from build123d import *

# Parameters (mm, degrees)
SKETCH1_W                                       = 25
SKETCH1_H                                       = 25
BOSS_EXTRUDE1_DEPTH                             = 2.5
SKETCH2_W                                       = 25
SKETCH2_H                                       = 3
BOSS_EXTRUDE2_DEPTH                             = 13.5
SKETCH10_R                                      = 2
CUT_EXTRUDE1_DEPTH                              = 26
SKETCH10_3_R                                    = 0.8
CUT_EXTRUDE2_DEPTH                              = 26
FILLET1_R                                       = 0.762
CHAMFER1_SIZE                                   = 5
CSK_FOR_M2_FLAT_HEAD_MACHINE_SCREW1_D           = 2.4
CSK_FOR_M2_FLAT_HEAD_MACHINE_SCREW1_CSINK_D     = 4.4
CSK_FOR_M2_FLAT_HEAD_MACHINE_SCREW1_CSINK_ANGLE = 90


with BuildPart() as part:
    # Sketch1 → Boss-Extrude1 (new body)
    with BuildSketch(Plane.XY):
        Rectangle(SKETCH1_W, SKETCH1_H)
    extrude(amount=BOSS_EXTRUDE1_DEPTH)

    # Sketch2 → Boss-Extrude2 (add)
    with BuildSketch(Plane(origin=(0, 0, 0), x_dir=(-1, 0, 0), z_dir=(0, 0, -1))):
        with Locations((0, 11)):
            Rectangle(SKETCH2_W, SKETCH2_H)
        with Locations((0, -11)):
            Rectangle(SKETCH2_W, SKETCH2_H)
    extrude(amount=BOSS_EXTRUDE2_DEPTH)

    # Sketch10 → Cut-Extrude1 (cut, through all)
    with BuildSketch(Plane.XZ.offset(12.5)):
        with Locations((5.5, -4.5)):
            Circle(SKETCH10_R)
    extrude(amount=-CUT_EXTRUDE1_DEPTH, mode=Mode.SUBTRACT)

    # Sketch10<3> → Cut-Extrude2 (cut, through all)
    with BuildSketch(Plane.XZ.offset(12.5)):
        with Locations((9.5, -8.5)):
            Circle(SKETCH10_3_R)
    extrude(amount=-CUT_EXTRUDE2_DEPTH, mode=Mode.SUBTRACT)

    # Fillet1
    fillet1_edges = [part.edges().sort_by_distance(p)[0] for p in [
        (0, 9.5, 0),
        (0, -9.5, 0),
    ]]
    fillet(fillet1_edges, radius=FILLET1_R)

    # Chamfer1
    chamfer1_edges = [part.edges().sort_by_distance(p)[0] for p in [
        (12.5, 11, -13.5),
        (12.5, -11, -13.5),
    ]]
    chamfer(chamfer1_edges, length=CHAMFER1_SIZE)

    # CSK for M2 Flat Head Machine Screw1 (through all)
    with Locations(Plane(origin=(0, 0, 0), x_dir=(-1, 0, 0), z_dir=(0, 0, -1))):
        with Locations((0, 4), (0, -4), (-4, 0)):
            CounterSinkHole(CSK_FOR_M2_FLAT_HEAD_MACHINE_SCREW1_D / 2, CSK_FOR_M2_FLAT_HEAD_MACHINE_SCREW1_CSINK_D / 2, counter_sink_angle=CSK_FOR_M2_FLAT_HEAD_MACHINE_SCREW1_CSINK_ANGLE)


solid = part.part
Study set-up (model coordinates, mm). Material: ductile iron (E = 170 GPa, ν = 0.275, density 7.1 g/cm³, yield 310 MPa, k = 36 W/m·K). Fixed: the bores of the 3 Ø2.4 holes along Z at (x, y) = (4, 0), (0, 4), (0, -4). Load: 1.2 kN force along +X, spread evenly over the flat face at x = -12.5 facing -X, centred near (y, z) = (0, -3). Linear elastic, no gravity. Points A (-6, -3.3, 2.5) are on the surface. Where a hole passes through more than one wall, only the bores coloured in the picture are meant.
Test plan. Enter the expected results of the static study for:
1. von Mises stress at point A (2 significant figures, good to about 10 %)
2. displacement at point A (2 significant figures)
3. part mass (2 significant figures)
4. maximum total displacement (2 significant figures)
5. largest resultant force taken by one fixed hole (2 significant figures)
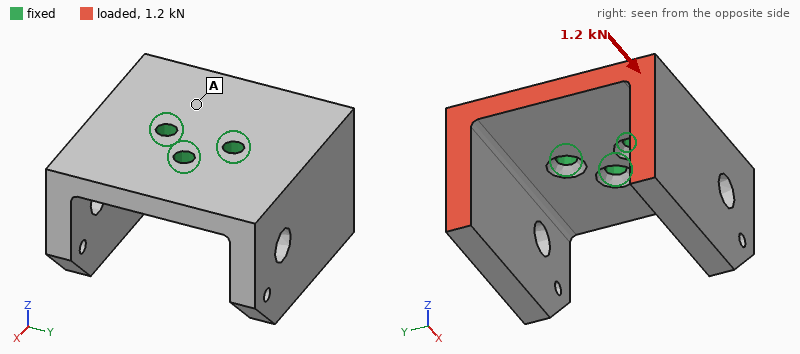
31 MPa
11 µm
24 g
52 µm
600 N
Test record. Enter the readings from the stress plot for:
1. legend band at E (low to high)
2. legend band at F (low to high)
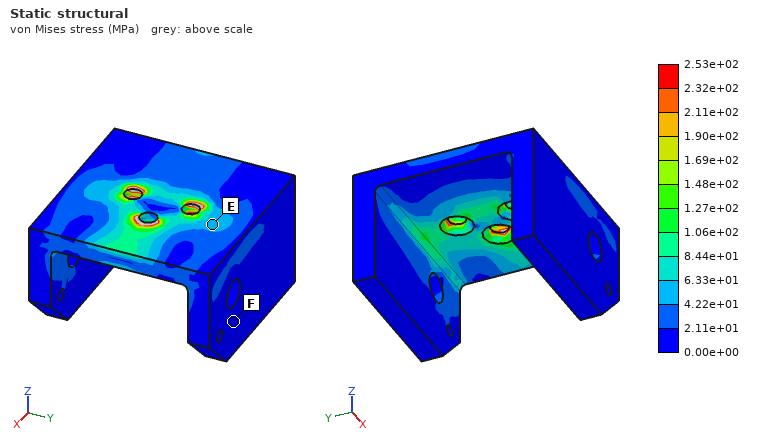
4.22e+01 to 6.33e+01 MPa
0.00e+00 to 2.11e+01 MPa
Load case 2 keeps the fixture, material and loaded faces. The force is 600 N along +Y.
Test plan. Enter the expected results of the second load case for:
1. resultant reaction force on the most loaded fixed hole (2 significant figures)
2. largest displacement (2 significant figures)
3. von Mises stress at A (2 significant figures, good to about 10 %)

790 N
59 µm
31 MPa
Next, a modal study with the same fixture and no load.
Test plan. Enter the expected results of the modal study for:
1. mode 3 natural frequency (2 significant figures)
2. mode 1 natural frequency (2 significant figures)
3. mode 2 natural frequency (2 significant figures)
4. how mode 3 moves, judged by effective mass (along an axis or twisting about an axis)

5100 Hz
4500 Hz
4600 Hz
along X
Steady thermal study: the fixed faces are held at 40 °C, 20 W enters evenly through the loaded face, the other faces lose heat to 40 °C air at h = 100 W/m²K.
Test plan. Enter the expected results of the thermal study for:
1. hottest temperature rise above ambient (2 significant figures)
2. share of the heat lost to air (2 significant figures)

67 K
41 %
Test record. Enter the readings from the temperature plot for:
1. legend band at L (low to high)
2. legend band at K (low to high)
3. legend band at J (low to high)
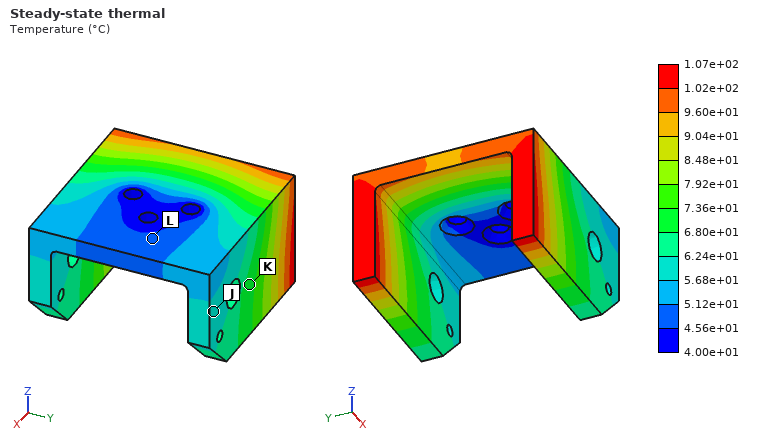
4.56e+01 to 5.12e+01 °C
6.80e+01 to 7.36e+01 °C
5.68e+01 to 6.24e+01 °C
